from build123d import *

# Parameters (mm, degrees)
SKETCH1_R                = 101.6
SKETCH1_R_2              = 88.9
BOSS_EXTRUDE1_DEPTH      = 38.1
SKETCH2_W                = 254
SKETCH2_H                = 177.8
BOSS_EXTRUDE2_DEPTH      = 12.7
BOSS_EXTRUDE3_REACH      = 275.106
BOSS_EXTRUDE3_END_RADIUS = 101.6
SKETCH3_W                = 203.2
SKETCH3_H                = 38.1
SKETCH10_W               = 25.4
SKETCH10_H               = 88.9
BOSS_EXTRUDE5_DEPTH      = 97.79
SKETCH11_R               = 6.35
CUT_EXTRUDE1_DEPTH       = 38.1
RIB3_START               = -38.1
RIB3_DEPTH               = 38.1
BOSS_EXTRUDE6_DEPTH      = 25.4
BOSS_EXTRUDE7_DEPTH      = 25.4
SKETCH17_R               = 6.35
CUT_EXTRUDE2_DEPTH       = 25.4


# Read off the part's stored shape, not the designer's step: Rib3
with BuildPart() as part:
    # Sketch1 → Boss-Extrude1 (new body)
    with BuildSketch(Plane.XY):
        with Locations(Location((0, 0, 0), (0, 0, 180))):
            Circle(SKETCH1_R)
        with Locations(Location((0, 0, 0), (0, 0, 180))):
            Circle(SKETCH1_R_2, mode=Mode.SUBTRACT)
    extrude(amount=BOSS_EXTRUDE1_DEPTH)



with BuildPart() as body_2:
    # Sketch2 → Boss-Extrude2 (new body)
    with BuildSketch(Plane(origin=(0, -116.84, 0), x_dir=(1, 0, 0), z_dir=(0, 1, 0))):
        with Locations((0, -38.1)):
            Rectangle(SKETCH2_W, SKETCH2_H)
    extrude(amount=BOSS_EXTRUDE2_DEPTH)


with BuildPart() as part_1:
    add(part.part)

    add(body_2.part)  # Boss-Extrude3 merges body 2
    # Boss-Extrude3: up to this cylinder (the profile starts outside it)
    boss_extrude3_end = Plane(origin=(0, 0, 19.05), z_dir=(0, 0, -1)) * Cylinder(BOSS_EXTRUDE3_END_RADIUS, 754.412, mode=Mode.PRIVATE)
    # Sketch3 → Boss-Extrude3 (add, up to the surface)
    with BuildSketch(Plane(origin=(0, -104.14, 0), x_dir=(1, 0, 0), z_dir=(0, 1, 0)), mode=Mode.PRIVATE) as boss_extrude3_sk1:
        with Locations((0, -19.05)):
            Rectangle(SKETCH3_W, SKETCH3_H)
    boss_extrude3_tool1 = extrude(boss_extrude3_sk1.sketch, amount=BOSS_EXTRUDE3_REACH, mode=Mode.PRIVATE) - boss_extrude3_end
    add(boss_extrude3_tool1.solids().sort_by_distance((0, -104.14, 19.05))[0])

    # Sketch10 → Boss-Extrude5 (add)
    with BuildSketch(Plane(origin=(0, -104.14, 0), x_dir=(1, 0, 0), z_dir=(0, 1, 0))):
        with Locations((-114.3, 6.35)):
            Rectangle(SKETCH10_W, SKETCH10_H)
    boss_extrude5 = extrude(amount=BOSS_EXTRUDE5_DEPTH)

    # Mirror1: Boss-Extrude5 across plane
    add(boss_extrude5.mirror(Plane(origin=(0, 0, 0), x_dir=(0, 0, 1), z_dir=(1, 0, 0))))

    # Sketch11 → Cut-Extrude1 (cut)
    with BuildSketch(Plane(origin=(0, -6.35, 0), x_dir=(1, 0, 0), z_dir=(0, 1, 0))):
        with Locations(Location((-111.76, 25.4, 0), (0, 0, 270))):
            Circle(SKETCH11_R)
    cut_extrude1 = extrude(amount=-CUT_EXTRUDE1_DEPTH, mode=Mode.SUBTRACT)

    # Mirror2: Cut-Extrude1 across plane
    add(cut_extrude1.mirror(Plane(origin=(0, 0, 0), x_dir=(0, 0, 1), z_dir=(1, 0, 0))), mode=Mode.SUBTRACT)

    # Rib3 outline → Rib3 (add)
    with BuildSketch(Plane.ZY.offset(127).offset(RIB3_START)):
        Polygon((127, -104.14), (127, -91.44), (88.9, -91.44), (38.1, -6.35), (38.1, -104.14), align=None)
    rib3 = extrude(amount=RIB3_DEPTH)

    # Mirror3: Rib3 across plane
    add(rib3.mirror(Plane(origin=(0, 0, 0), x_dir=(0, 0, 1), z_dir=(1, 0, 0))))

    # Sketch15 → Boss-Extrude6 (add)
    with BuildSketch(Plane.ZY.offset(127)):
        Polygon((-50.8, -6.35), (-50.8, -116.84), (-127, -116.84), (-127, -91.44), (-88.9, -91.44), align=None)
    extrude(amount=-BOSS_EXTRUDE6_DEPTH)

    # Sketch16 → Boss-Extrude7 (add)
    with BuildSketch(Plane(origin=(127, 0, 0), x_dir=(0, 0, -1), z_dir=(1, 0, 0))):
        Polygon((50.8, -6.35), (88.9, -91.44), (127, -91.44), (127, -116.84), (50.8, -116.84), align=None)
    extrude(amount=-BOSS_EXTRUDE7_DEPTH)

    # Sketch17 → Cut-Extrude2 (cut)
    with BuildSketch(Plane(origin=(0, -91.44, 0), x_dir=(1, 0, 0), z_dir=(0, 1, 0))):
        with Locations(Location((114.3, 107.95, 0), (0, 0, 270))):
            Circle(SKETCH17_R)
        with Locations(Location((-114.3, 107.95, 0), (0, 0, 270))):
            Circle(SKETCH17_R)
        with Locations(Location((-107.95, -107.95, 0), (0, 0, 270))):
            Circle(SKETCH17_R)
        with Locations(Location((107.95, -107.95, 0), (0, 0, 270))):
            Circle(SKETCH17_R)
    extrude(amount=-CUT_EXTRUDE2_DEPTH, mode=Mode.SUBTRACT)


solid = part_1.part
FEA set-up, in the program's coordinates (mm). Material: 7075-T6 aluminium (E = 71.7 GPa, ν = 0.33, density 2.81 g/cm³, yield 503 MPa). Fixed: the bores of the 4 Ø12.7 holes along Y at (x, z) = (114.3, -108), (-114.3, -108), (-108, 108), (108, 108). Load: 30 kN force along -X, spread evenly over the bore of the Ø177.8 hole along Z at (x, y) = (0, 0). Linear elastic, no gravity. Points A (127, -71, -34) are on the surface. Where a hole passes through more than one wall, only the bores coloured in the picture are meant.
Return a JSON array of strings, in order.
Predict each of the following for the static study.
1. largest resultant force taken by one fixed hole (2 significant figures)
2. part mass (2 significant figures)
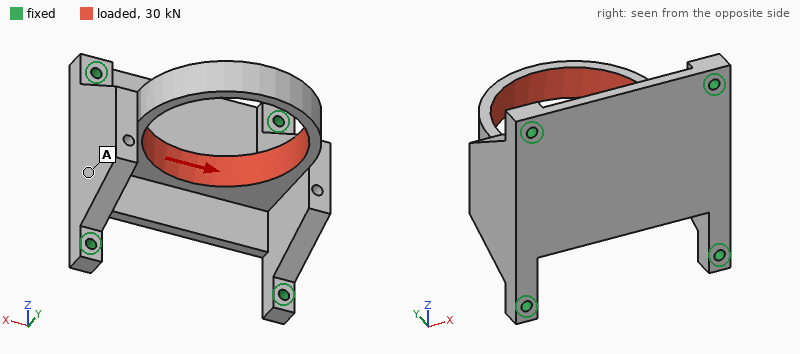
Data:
["19 kN", "5.3 kg"]
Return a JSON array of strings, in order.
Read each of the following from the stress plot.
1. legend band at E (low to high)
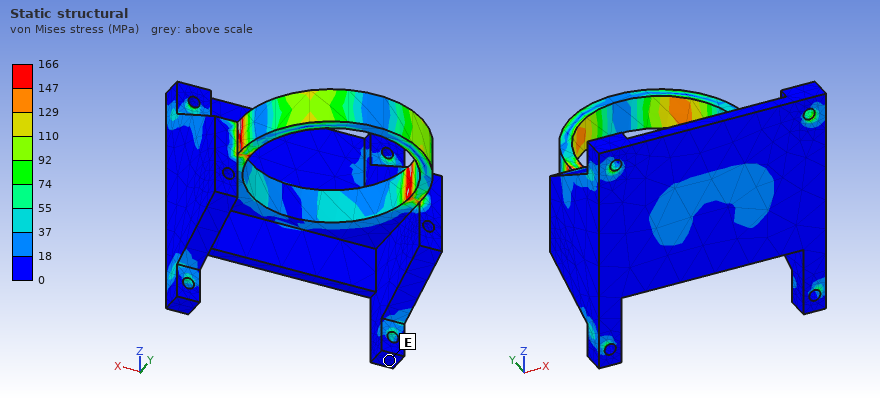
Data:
["0 to 18 MPa"]
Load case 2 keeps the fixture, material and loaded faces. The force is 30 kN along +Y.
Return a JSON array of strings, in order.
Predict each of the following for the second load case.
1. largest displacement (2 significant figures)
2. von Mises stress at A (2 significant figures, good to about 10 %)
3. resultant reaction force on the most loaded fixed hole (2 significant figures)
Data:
["0.12 mm", "5.5 MPa", "10 kN"]
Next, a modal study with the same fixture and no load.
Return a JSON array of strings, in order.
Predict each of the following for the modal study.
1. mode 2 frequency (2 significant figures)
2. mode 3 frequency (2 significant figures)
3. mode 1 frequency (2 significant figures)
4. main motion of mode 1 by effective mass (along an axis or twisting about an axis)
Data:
["1100 Hz", "1200 Hz", "1000 Hz", "along X"]
